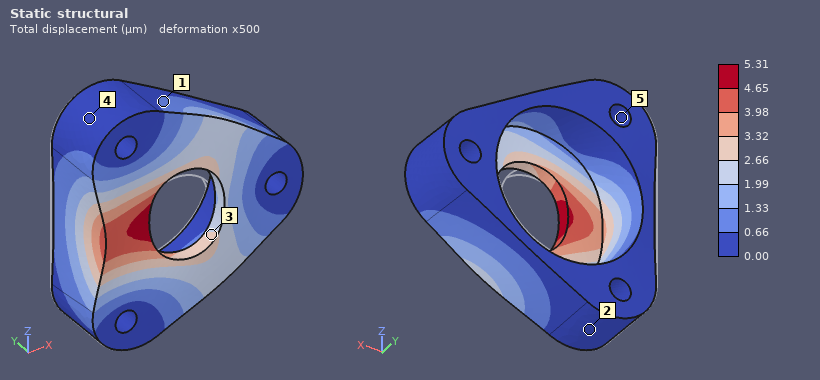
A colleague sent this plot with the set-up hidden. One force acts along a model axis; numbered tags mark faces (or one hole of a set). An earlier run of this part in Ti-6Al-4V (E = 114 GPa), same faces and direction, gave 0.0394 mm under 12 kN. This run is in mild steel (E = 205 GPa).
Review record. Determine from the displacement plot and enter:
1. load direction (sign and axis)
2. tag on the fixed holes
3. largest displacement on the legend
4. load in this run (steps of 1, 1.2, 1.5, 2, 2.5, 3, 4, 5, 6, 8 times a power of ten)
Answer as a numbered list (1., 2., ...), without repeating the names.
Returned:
1. +X
2. 5
3. 5.31 µm
4. 3 kN
